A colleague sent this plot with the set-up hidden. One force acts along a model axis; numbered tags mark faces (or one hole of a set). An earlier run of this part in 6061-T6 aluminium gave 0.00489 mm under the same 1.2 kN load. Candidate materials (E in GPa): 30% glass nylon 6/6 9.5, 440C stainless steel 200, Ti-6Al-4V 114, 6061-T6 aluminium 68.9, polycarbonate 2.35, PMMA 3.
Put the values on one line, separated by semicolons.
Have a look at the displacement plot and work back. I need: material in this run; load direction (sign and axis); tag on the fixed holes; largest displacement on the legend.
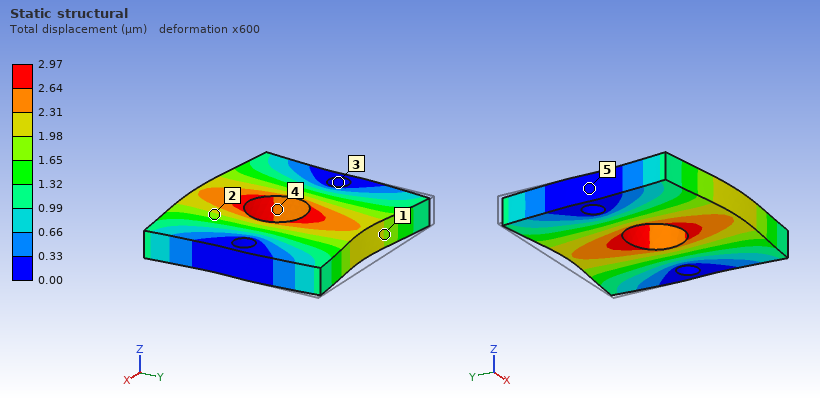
Ti-6Al-4V; -Y; 3; 2.97 µm
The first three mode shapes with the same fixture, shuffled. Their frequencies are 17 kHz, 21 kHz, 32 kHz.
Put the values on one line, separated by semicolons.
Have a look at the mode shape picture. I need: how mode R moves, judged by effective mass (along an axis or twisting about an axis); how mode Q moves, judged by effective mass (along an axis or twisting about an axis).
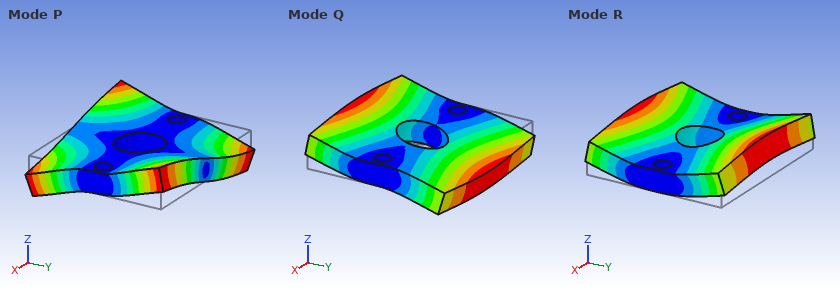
along Z; twisting about X
